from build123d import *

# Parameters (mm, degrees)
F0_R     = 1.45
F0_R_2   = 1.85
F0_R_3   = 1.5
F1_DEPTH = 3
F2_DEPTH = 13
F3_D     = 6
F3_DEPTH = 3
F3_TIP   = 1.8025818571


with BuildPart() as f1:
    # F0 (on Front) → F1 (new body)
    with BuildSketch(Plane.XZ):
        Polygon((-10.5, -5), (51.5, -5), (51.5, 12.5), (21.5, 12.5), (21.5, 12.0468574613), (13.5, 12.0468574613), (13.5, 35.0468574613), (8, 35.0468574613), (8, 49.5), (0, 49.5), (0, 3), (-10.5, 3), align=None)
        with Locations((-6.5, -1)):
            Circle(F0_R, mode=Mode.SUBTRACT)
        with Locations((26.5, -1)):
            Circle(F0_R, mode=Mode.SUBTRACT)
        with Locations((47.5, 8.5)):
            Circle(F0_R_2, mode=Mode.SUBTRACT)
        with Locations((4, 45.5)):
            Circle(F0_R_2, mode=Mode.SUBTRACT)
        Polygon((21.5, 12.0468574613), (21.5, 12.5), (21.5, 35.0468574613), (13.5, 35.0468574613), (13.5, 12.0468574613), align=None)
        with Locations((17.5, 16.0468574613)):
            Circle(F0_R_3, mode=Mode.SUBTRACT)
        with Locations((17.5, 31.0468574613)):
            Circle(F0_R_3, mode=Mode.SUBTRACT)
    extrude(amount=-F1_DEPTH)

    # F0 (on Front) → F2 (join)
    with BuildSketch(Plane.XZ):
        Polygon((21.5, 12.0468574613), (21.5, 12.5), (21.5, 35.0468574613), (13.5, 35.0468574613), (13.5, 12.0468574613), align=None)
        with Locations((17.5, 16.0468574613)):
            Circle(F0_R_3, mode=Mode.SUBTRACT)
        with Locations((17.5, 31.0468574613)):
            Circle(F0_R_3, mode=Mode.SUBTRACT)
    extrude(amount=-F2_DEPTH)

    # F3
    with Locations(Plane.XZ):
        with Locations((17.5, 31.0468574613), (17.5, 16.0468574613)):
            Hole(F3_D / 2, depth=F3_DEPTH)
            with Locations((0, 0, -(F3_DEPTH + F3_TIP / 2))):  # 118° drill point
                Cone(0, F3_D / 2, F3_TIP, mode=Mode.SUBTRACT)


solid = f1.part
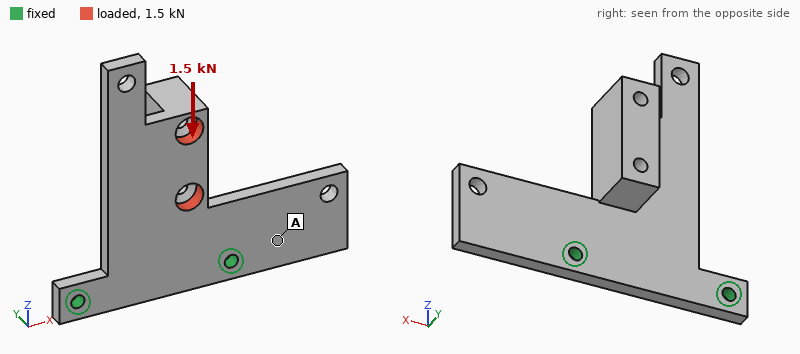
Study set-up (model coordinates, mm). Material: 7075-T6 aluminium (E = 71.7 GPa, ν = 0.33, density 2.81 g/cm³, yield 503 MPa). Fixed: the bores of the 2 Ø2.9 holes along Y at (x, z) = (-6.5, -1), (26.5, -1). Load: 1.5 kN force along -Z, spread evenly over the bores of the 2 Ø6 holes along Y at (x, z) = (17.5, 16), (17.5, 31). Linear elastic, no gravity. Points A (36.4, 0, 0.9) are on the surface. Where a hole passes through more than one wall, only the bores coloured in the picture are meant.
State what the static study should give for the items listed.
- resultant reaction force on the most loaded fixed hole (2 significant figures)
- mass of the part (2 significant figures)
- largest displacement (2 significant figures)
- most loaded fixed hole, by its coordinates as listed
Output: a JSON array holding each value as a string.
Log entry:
["1.1 kN", "17 g", "57 µm", "(26.5, -1)"]
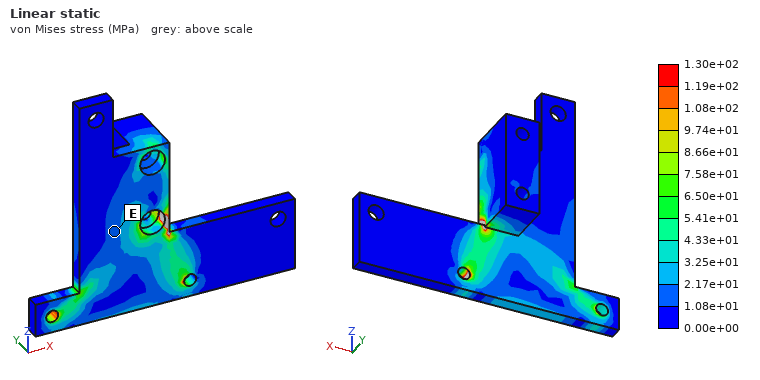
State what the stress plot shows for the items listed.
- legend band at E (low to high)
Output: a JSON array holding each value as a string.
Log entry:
["1.08e+01 to 2.17e+01 MPa"]
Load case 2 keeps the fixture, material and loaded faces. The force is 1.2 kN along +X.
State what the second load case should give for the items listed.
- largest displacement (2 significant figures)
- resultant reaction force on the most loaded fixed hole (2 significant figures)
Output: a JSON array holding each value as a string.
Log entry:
["0.13 mm", "1.2 kN"]
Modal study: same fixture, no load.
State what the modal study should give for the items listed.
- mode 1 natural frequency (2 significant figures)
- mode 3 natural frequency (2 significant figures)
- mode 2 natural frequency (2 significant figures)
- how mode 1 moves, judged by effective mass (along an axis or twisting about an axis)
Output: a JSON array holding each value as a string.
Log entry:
["1100 Hz", "4400 Hz", "3700 Hz", "along Y"]
